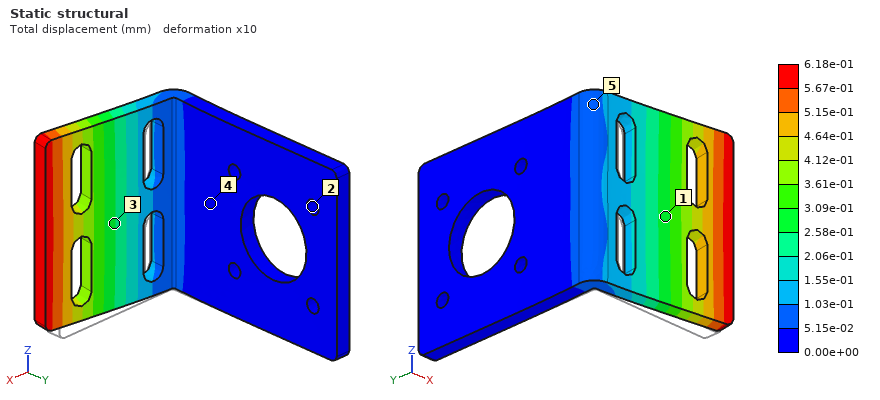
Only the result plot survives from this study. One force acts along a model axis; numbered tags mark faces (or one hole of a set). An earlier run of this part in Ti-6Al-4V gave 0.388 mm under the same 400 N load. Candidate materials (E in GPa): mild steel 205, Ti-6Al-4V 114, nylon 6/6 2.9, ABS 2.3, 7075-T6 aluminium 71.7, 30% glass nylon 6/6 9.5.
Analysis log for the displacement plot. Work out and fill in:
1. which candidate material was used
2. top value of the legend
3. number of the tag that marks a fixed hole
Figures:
7075-T6 aluminium
6.18e-01 mm
2
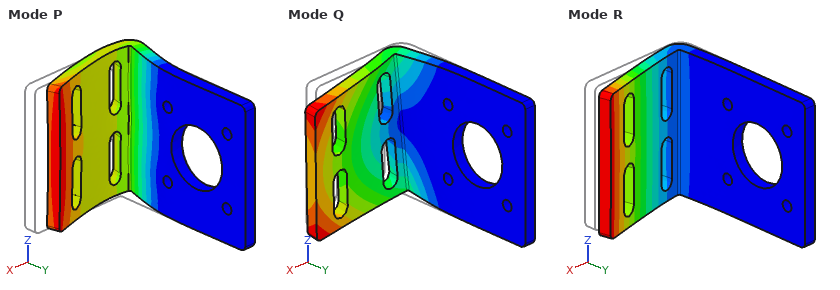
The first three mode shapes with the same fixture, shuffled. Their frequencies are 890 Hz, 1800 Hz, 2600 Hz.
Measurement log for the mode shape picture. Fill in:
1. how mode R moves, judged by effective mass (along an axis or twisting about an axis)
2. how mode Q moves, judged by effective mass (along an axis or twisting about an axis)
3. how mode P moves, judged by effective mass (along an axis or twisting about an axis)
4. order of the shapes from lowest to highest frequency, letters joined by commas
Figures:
along Y
along Z
along X
R, Q, P
